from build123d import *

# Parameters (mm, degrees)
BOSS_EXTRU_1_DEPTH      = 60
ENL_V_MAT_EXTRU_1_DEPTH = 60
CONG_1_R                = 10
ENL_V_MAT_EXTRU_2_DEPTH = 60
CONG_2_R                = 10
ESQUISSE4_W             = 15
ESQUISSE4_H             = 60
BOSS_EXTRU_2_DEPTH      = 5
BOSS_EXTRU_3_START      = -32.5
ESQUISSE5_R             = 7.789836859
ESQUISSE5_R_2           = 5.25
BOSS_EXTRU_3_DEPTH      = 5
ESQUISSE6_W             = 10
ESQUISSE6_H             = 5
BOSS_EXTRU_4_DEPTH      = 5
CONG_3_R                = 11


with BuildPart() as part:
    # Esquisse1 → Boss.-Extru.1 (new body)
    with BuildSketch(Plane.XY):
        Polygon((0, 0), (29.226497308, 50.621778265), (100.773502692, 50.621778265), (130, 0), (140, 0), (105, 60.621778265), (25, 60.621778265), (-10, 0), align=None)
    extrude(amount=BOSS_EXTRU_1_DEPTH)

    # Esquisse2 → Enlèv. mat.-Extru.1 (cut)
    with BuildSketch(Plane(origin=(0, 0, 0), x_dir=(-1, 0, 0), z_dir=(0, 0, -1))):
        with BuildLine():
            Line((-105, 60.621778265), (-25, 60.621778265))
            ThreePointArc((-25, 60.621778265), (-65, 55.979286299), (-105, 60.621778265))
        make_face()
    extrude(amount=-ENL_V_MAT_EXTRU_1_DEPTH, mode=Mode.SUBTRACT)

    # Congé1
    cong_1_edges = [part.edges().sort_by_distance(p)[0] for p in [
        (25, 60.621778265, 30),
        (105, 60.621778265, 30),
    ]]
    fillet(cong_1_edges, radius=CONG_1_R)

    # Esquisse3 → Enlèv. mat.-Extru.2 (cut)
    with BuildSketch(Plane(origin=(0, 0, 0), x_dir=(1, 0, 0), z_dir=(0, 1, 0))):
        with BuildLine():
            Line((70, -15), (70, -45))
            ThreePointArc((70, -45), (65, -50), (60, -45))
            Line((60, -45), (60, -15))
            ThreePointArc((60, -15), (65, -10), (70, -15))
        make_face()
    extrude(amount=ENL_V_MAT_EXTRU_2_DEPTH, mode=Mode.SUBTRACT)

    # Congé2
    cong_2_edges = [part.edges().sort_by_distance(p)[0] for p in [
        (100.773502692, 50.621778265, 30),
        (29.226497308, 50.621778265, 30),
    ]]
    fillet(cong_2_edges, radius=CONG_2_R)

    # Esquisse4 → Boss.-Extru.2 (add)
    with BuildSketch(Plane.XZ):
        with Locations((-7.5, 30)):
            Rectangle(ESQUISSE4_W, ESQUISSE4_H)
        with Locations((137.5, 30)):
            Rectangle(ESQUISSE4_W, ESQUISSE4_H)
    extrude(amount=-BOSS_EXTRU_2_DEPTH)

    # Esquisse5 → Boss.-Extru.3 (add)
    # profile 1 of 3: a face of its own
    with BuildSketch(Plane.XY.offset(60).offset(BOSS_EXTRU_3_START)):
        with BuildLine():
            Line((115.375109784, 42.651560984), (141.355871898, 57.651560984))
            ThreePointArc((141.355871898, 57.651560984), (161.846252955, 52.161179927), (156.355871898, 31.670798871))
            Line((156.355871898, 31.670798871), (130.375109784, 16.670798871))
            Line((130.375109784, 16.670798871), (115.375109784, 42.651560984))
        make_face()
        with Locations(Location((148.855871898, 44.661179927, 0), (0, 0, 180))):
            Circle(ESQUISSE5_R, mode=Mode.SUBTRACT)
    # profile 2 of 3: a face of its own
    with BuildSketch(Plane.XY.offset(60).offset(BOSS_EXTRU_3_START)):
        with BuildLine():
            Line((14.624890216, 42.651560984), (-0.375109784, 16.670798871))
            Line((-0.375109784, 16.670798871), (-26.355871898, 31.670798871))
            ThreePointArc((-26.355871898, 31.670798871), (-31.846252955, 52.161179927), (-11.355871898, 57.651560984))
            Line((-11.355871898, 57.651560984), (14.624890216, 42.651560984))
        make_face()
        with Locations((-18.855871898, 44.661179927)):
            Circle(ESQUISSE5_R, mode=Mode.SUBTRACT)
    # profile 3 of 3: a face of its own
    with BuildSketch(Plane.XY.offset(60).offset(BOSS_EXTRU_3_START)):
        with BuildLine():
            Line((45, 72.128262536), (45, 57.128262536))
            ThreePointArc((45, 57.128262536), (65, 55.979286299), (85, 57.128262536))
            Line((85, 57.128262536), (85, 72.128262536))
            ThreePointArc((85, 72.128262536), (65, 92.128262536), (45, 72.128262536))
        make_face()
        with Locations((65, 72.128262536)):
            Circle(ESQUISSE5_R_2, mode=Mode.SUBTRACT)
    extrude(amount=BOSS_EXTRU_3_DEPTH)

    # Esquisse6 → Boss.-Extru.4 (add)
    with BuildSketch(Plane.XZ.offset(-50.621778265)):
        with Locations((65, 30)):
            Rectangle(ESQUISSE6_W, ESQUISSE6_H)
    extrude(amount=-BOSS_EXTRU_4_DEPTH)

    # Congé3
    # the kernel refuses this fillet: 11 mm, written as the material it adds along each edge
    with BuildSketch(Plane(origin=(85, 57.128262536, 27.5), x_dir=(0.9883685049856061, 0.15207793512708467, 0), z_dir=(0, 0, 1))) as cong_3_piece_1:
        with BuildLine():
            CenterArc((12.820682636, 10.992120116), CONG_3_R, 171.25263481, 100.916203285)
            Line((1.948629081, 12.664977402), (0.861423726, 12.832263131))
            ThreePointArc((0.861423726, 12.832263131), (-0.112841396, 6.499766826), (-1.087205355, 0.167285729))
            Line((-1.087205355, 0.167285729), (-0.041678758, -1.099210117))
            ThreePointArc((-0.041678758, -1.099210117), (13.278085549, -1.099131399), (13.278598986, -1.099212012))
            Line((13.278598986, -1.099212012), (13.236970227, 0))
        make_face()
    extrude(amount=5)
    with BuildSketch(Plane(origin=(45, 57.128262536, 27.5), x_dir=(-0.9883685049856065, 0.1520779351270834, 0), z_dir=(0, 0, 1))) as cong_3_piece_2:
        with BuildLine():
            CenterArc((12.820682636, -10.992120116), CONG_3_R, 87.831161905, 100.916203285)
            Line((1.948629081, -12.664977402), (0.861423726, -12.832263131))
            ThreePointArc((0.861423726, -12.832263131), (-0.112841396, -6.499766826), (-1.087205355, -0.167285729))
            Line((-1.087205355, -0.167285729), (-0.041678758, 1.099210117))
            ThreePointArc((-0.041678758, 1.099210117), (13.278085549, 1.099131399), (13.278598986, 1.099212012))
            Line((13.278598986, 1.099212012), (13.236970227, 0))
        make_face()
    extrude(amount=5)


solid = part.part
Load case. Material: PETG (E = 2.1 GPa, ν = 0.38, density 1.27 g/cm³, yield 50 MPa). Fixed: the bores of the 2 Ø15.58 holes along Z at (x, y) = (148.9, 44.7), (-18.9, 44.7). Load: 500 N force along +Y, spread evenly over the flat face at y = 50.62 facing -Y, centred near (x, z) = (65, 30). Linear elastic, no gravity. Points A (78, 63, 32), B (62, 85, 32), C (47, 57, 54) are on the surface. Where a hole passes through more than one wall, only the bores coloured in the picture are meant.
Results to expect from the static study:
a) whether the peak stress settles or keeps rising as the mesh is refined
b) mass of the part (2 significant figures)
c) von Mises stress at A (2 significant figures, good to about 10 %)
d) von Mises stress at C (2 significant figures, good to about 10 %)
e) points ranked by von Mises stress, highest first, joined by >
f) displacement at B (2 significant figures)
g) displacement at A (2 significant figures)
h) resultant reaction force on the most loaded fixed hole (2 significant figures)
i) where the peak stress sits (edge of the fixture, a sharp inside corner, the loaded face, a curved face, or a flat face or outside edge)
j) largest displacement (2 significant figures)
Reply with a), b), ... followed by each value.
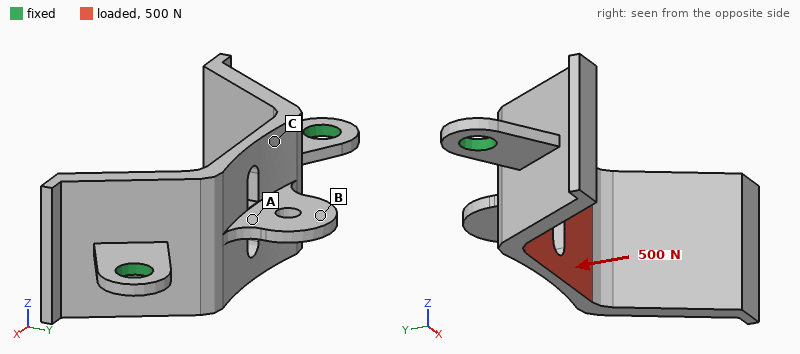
a) keeps rising
b) 150 g
c) 4.2 MPa
d) 2.4 MPa
e) A > C > B
f) 0.50 mm
g) 0.51 mm
h) 420 N
i) edge of the fixture
j) 0.71 mm
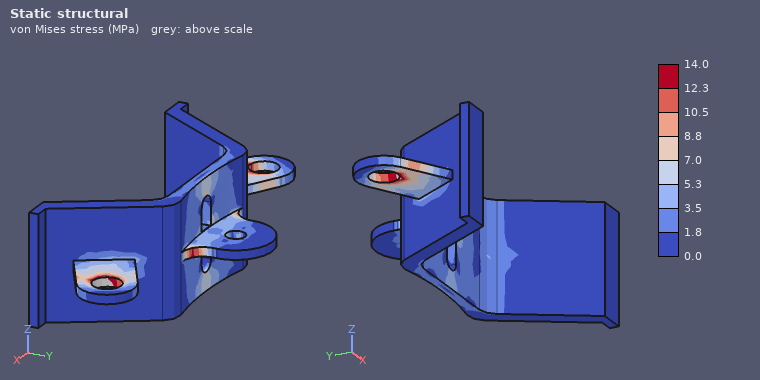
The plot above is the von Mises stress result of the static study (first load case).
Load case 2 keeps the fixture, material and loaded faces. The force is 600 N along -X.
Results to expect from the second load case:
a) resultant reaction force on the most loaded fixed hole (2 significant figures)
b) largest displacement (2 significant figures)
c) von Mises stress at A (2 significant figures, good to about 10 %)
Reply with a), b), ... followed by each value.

a) 300 N
b) 0.20 mm
c) 0.93 MPa
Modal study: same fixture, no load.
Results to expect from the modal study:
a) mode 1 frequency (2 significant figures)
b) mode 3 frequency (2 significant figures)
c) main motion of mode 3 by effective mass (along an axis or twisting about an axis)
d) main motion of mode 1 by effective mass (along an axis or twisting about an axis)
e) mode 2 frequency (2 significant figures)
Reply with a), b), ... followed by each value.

a) 160 Hz
b) 370 Hz
c) along Z
d) twisting about X
e) 330 Hz
